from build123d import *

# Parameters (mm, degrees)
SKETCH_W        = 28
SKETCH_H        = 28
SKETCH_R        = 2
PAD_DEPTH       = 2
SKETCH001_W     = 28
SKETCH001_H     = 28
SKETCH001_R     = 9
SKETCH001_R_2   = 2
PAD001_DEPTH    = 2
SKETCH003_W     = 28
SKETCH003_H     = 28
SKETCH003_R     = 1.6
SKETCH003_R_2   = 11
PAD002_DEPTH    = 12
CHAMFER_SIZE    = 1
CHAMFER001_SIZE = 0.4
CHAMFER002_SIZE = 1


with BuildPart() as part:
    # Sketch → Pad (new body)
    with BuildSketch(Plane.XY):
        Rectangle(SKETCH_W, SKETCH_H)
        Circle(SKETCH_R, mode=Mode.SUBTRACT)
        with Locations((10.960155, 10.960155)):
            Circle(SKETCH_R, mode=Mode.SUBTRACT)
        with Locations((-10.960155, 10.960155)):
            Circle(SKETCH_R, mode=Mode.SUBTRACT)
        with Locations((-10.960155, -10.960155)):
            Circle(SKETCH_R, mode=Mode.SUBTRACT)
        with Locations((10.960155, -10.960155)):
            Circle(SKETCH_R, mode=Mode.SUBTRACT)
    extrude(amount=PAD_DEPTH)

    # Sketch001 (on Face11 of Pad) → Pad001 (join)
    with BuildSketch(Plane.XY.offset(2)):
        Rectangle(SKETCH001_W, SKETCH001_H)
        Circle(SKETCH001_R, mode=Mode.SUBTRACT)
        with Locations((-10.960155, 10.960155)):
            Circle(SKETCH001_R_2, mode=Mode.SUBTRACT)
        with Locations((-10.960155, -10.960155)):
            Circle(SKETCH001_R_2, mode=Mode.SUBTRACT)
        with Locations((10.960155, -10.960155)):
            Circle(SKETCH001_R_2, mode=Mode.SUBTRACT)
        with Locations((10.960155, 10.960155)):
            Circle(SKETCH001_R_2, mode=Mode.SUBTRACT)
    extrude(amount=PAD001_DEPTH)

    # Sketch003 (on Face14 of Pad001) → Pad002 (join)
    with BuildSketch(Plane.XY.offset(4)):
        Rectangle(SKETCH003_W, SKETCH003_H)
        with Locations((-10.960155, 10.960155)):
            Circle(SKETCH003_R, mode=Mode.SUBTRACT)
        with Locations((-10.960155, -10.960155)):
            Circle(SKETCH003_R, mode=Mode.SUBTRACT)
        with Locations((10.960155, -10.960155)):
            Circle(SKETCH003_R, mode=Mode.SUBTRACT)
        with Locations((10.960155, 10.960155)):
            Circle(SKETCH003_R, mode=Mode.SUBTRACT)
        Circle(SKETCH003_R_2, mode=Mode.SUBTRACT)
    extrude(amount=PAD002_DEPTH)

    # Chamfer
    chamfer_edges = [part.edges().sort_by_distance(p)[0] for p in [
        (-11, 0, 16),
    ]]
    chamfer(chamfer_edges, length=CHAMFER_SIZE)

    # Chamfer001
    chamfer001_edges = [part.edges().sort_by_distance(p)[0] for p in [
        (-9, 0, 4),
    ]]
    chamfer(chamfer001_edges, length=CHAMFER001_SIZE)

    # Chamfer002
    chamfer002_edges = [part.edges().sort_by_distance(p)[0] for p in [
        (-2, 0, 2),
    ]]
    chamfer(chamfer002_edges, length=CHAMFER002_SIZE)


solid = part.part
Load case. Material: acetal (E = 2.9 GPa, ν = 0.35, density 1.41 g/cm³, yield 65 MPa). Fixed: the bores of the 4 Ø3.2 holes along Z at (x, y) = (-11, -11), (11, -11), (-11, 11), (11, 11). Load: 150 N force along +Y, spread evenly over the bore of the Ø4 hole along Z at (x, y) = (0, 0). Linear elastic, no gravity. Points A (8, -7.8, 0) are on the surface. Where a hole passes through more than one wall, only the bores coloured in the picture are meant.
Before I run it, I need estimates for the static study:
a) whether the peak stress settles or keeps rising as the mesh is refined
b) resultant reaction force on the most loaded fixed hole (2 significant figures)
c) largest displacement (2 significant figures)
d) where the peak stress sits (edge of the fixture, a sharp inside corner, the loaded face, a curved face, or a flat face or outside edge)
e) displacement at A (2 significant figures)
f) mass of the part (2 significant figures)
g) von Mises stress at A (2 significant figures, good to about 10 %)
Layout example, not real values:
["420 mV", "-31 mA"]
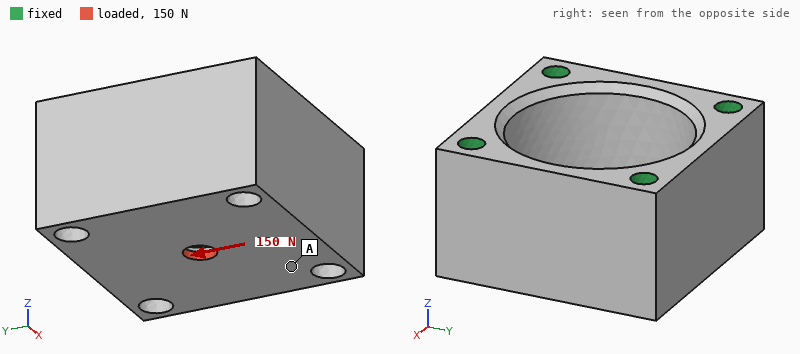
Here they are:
["keeps rising", "42 N", "24 µm", "a sharp inside corner", "6.0 µm", "9.6 g", "1.4 MPa"]
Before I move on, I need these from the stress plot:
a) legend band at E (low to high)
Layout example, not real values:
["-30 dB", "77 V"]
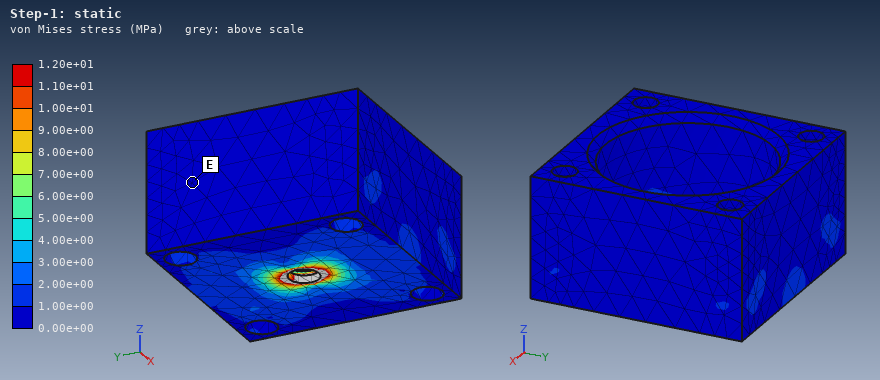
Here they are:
["0.00e+00 to 1.00e+00 MPa"]
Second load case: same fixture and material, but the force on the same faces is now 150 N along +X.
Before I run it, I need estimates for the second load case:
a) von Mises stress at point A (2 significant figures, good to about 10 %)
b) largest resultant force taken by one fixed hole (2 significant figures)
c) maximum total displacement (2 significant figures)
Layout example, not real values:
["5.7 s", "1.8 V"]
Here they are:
["1.4 MPa", "42 N", "24 µm"]
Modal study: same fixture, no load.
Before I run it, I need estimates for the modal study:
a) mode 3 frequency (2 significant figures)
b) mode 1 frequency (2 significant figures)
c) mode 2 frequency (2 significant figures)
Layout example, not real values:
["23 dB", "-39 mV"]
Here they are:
["15 kHz", "12 kHz", "15 kHz"]
